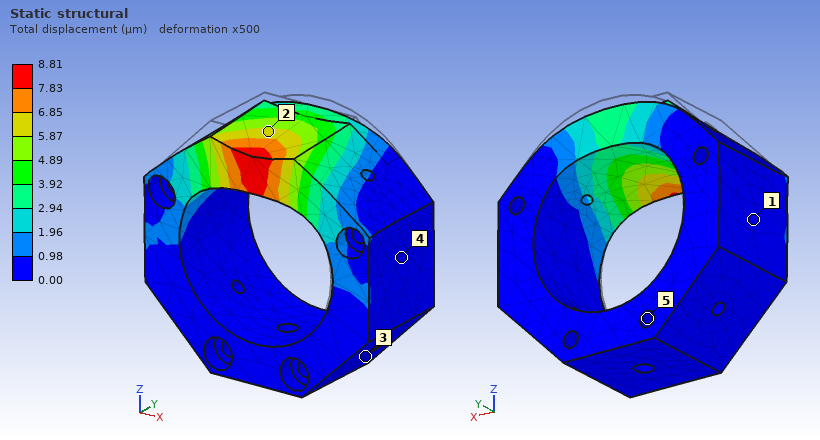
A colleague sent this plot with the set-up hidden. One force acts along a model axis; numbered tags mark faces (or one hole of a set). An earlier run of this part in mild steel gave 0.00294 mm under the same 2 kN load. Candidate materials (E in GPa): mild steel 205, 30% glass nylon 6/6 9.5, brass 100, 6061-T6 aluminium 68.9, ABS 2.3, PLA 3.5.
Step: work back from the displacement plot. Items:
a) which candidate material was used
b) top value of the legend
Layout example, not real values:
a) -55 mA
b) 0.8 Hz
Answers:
a) 6061-T6 aluminium
b) 8.81 µm
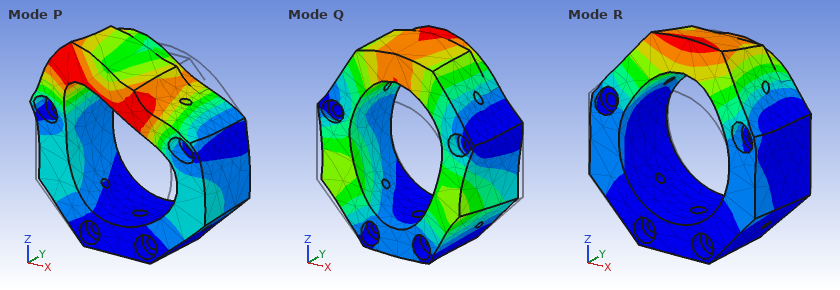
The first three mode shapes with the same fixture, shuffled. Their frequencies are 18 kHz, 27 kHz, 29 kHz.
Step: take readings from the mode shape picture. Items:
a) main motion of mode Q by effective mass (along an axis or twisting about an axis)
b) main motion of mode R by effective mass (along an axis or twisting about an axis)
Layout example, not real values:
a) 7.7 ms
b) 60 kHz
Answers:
a) along Z
b) along Y
